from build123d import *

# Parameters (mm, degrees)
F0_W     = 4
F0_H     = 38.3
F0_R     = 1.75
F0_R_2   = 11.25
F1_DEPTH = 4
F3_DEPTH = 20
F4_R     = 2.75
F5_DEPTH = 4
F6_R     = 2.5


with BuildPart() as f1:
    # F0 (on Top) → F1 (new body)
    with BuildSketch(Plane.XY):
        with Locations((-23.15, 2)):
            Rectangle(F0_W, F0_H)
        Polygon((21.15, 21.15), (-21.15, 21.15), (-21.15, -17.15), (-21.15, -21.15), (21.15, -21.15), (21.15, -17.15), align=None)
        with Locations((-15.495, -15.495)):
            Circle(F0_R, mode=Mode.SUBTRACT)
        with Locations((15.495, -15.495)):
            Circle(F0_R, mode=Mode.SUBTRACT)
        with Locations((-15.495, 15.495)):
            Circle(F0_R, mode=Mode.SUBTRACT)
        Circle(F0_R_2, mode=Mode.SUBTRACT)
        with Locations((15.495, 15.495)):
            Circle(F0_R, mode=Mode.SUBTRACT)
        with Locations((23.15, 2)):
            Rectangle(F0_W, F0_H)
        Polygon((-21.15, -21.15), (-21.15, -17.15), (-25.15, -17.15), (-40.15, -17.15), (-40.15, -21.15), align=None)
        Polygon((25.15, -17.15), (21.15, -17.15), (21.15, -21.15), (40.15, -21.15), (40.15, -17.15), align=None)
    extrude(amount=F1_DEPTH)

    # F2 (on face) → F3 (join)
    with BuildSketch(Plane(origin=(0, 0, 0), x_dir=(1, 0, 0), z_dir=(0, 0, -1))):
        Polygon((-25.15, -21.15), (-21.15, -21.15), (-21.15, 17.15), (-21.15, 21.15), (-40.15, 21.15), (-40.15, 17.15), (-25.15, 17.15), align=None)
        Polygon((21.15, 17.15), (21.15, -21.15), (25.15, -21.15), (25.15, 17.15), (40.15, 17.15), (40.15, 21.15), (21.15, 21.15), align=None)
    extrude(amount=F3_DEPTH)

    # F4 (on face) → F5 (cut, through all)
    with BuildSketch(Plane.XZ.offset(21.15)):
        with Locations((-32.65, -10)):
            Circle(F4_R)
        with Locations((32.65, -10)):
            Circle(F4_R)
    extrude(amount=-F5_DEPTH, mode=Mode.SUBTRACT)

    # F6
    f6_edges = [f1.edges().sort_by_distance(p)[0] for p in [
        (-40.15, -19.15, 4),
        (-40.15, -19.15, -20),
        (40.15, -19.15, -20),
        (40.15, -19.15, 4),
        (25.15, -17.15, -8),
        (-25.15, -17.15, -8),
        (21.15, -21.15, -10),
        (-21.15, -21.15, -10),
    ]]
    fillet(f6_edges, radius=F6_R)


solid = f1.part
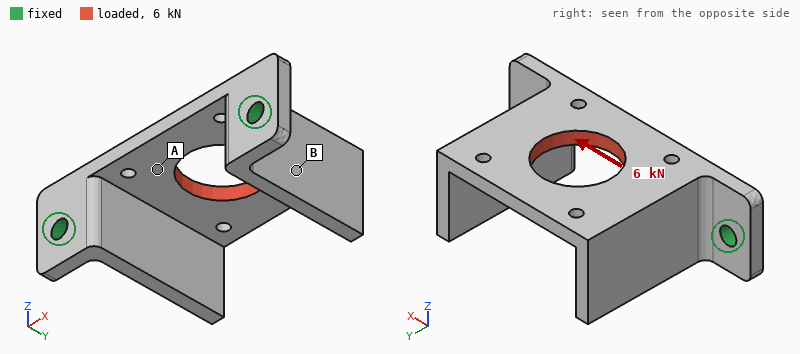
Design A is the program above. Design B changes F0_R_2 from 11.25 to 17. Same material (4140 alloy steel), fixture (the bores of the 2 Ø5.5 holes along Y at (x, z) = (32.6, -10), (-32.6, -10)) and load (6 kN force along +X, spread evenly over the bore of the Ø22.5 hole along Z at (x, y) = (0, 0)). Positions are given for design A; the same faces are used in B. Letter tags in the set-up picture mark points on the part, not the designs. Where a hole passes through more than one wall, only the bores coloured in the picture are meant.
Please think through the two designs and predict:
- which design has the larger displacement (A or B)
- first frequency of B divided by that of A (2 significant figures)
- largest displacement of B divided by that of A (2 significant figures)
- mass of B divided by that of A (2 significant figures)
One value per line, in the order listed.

B
1.1
1.6
0.87
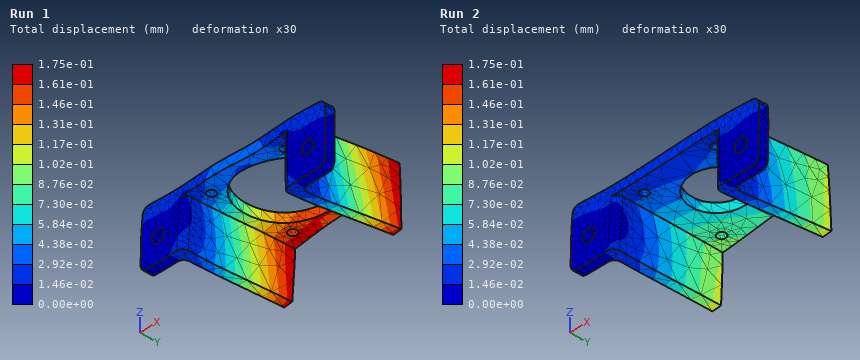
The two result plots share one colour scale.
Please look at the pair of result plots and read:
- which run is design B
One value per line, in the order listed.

Run 1
